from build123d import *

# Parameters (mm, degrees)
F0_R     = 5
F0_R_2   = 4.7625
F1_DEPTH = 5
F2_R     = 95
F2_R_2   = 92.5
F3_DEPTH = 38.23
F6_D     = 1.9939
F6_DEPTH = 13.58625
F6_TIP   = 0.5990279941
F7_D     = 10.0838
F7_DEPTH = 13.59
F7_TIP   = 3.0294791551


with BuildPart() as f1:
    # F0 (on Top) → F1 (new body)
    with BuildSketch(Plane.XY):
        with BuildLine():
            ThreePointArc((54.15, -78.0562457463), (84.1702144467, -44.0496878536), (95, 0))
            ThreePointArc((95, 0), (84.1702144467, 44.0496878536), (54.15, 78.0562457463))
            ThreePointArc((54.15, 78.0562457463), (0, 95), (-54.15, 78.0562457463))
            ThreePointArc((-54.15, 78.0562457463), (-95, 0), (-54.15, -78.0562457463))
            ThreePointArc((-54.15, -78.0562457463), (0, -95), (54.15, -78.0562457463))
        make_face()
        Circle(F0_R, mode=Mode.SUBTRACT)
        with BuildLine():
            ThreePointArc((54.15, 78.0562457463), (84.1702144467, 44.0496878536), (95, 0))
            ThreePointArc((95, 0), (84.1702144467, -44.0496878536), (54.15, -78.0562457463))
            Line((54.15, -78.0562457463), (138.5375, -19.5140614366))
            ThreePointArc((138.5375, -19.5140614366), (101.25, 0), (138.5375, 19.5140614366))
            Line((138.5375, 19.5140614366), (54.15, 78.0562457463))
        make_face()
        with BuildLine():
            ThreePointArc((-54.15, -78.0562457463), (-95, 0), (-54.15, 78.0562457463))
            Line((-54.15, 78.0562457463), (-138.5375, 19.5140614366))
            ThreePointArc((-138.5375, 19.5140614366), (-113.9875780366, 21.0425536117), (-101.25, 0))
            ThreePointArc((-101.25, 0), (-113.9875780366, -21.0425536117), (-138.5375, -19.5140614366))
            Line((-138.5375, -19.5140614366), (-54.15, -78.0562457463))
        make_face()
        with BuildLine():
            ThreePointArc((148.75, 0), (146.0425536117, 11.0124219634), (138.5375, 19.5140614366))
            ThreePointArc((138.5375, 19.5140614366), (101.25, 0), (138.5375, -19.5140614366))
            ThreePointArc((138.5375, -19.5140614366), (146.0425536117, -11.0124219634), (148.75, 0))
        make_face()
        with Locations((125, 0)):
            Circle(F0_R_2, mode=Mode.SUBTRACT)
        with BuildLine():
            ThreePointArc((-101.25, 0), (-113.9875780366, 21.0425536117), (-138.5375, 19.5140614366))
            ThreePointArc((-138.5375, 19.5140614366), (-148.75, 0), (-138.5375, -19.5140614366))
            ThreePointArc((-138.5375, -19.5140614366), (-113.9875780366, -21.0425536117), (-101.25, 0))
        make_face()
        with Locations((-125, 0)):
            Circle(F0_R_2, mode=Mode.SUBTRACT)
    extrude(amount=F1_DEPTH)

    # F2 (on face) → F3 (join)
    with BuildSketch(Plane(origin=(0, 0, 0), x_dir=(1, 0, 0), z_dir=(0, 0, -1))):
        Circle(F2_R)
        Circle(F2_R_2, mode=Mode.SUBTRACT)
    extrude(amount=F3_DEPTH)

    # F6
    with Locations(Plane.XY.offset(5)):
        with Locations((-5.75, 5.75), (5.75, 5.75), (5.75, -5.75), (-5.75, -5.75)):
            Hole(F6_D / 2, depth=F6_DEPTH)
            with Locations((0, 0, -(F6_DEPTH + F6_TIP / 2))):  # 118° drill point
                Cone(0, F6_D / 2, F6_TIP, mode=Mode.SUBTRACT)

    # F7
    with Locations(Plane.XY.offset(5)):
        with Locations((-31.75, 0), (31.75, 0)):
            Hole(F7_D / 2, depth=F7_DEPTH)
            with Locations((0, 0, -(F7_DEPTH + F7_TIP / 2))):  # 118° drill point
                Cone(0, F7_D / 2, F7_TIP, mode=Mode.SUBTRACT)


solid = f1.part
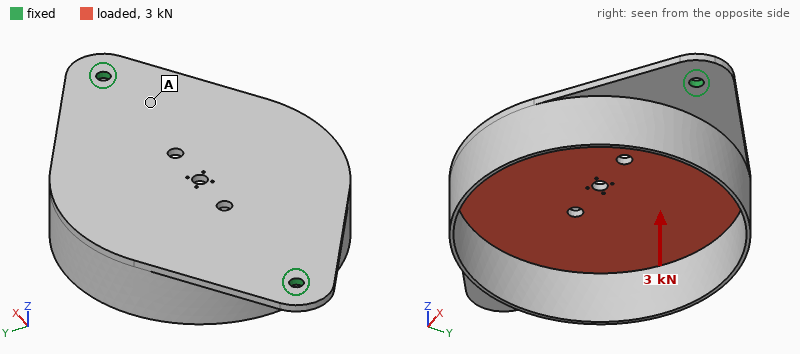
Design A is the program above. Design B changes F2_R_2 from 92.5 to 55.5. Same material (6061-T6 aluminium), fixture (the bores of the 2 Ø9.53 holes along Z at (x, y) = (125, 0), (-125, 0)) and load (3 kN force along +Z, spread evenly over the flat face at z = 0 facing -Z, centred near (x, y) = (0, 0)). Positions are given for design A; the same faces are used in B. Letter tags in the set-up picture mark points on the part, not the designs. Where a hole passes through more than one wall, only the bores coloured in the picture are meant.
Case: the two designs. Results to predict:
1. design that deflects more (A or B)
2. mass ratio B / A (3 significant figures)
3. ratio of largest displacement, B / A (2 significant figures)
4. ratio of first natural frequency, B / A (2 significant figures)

A
3.78
0.11
0.56
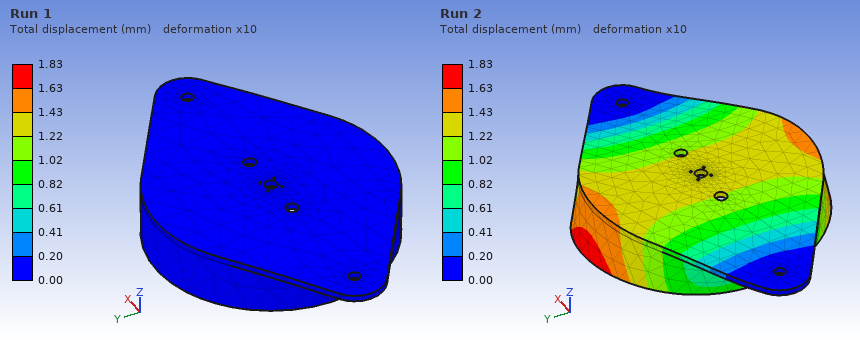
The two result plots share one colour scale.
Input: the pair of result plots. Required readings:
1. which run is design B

Run 1
